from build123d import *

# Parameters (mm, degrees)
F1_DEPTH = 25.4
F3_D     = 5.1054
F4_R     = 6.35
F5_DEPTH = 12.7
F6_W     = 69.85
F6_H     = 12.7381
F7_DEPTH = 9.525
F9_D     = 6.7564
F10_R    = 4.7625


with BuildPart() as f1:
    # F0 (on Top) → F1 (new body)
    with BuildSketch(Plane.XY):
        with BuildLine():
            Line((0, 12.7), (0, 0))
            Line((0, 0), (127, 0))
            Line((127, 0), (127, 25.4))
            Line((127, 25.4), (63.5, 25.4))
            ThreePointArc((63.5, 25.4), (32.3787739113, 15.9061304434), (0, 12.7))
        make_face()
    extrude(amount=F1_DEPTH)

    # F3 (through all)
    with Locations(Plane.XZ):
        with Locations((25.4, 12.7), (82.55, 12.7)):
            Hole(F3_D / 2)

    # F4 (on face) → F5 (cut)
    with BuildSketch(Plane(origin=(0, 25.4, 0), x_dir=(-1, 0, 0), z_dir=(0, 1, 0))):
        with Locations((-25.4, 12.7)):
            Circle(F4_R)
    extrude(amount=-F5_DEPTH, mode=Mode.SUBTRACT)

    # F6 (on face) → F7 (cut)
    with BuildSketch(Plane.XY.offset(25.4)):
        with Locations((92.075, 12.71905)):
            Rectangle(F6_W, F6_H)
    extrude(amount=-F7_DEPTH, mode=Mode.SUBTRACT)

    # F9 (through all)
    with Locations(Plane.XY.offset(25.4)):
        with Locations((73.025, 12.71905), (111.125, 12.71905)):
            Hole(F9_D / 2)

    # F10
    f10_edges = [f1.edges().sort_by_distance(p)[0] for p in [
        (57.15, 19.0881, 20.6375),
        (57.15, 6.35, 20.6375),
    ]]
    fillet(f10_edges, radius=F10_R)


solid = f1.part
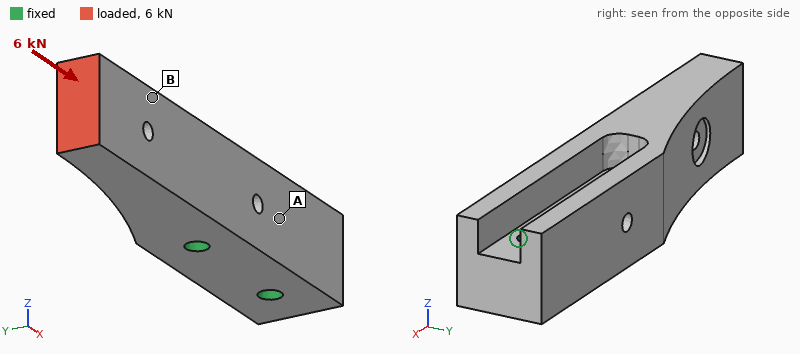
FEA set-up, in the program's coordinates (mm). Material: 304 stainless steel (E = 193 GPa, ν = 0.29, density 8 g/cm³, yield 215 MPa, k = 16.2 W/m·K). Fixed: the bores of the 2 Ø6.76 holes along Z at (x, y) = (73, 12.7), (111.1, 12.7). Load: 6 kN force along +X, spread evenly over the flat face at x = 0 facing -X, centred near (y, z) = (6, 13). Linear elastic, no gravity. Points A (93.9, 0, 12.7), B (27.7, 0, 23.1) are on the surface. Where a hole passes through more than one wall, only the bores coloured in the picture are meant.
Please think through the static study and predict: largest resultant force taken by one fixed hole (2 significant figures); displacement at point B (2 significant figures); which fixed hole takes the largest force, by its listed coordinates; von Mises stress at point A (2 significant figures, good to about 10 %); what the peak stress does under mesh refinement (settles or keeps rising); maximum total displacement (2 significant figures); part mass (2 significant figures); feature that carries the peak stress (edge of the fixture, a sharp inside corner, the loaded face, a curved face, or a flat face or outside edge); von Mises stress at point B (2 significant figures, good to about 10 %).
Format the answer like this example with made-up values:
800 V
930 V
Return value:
5.0 kN
14 µm
(73, 12.7)
6.9 MPa
keeps rising
25 µm
460 g
edge of the fixture
23 MPa
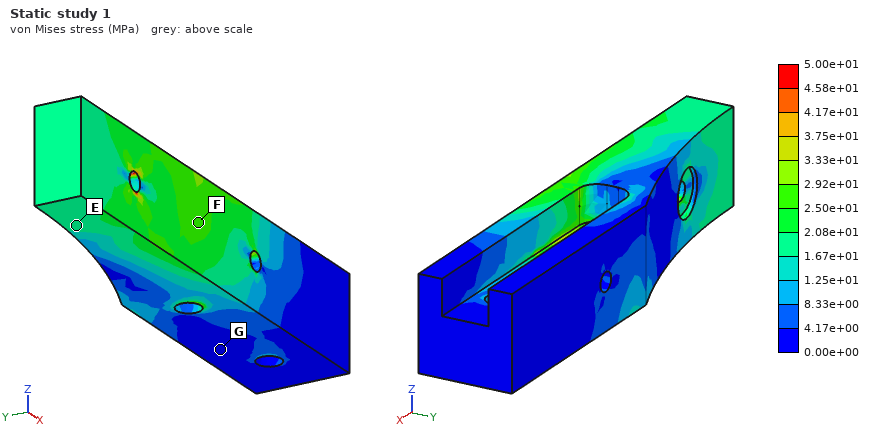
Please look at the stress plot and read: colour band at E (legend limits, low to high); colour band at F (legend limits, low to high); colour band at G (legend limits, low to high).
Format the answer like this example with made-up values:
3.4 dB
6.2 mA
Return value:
1.67e+01 to 2.08e+01 MPa
2.50e+01 to 2.92e+01 MPa
0.00e+00 to 4.17e+00 MPa
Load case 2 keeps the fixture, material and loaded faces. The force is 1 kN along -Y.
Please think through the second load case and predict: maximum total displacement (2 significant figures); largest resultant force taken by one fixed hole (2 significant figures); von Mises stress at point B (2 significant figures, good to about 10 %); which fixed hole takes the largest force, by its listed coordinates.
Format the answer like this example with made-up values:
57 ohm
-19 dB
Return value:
57 µm
2.2 kN
35 MPa
(73, 12.7)
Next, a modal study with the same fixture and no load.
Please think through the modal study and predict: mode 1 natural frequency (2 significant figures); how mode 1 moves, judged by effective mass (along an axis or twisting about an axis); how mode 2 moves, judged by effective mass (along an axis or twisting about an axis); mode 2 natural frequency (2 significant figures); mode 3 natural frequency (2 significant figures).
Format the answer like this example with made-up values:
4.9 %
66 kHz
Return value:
3200 Hz
along Y
along Z
3400 Hz
9600 Hz
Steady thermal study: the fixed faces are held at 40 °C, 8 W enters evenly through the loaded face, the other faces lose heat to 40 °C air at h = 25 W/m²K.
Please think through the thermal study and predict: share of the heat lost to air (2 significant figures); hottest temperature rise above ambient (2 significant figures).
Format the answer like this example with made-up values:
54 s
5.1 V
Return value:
51 %
64 K
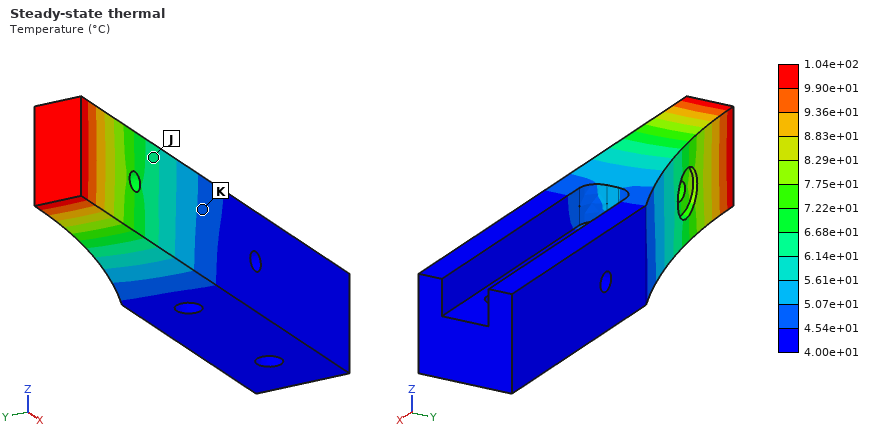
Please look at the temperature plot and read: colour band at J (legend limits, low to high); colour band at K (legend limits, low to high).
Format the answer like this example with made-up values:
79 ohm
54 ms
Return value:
6.14e+01 to 6.68e+01 °C
4.54e+01 to 5.07e+01 °C
